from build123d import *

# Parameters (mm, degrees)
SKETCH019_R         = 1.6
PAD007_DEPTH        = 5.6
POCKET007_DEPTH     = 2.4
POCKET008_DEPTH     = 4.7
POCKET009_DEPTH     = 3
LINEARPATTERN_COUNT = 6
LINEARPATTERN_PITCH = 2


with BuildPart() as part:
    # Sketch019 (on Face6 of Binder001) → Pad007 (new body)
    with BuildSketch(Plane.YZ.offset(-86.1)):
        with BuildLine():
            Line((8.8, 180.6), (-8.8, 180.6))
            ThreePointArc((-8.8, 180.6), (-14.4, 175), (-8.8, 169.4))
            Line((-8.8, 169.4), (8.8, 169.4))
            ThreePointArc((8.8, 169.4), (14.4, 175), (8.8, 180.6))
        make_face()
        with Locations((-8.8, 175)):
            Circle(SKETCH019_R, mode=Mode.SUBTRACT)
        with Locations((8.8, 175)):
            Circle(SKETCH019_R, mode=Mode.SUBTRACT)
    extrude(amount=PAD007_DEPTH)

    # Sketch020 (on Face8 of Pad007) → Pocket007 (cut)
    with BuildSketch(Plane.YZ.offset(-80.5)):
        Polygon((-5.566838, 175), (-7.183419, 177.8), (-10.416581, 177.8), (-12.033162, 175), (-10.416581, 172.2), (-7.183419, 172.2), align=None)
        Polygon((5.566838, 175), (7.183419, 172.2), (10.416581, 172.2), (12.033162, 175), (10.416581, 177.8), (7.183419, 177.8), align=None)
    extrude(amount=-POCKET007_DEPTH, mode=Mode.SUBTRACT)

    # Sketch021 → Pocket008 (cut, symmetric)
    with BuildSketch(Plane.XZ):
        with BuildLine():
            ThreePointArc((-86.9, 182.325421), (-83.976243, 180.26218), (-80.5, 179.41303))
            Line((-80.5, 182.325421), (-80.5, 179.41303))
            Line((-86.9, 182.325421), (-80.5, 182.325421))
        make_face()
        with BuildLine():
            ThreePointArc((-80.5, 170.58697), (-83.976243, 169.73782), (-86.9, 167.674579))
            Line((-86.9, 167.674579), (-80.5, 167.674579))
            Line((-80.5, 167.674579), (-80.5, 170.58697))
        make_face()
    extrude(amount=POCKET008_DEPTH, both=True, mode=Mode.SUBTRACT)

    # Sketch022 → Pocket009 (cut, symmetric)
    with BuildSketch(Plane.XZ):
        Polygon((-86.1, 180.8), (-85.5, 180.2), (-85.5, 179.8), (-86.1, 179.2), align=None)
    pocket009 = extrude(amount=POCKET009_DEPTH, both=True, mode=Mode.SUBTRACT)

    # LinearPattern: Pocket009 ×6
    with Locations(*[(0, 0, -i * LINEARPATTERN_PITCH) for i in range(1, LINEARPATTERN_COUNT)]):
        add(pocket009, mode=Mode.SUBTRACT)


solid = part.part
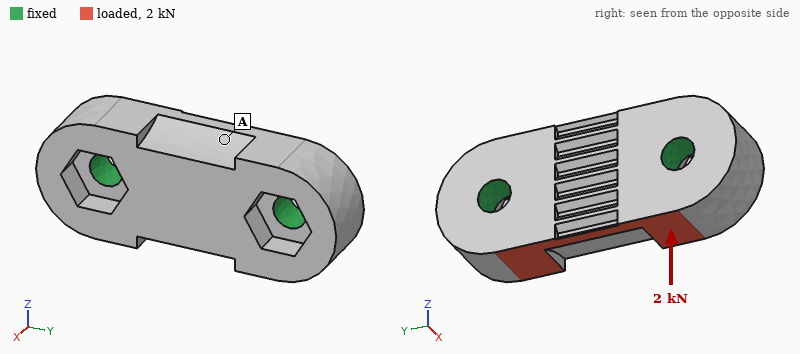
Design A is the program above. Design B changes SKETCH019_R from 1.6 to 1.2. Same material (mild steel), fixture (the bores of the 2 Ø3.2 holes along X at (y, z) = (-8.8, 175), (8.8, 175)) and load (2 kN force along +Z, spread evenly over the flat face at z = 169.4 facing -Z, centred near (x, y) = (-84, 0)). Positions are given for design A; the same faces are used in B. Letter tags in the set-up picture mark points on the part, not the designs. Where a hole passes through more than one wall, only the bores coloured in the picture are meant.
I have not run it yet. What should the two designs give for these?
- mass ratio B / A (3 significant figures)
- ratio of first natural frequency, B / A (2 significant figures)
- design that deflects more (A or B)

1.02
0.84
B
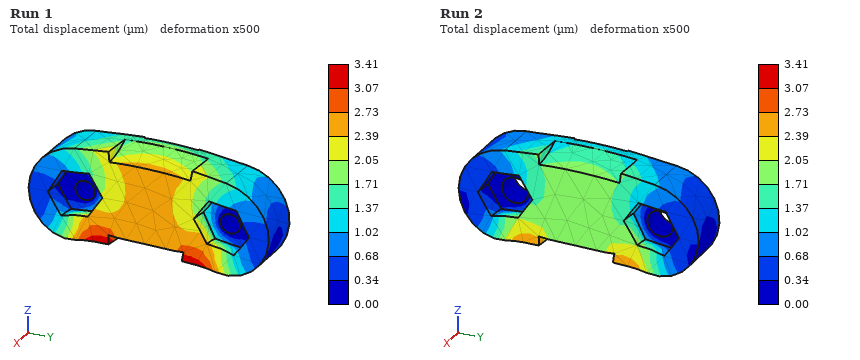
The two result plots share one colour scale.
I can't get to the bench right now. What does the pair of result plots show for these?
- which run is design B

Run 1
